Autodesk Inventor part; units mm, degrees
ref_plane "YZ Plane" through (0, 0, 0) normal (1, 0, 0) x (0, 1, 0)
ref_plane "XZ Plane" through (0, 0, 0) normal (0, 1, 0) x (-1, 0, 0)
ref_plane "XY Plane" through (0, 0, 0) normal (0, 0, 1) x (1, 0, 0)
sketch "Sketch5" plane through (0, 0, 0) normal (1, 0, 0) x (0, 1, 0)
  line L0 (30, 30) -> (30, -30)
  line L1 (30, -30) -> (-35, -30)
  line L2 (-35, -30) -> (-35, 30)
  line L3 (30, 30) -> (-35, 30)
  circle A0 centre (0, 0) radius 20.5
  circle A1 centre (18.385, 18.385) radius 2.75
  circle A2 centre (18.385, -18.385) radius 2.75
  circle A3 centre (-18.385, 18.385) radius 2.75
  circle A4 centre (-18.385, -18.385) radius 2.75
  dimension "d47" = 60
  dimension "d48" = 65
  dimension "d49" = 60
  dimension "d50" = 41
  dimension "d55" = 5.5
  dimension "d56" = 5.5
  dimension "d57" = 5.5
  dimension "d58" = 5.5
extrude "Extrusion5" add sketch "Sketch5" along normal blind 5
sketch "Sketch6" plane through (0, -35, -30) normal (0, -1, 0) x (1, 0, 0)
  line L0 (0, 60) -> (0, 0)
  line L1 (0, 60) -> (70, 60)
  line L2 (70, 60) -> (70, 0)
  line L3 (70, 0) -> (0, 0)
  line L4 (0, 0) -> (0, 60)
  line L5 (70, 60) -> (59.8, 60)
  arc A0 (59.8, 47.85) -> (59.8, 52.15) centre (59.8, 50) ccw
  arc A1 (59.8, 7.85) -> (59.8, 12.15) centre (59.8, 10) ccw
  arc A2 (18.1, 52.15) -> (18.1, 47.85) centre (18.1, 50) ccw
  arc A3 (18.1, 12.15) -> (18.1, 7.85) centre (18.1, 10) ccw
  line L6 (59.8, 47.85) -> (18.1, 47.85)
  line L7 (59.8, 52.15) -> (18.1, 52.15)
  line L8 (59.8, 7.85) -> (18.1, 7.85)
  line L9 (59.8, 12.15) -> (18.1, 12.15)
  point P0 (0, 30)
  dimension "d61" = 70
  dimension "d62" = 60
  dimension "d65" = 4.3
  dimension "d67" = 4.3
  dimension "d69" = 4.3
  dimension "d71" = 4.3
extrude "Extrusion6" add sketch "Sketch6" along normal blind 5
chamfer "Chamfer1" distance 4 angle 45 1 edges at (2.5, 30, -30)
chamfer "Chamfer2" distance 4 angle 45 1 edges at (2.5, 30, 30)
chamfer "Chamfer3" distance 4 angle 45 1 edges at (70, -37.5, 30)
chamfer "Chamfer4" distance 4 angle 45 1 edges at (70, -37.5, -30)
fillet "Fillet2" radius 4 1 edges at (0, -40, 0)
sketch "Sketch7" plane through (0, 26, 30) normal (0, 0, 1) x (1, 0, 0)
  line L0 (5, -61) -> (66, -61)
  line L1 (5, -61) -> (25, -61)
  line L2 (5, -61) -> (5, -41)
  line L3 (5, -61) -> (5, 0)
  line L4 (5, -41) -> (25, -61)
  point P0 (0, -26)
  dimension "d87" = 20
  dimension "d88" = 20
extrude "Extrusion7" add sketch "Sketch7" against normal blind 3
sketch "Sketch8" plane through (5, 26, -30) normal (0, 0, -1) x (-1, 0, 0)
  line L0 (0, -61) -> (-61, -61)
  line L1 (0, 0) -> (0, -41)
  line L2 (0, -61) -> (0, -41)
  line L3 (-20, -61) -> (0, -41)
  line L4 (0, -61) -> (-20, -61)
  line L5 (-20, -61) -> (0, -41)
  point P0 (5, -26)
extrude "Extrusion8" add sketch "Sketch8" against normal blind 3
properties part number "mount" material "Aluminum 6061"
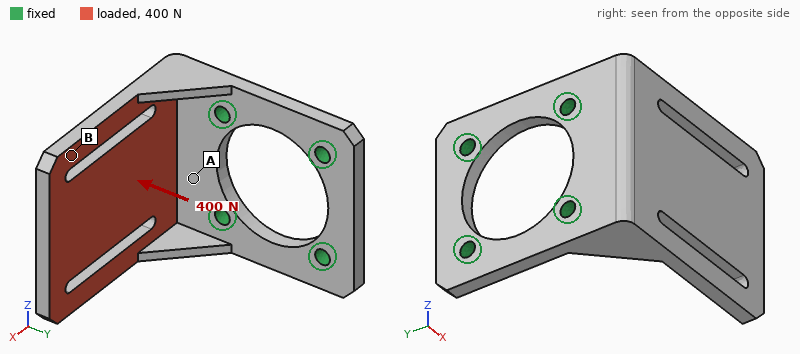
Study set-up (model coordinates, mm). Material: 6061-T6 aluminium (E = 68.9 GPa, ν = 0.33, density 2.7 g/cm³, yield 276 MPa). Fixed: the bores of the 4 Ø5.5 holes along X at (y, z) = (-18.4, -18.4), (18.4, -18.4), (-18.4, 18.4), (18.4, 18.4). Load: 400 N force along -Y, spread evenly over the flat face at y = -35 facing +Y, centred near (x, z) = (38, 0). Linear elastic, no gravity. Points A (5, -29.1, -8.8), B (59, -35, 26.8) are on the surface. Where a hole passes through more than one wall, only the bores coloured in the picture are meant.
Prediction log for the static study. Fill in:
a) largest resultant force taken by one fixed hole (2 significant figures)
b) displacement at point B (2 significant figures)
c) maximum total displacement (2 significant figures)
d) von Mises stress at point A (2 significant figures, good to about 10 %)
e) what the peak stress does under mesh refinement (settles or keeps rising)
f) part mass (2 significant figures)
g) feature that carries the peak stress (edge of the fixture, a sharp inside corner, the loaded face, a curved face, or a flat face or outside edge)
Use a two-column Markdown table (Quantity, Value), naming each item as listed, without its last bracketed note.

| Quantity | Value |
|---|---|
| largest resultant force taken by one fixed hole | 170 N |
| displacement at point B | 0.36 mm |
| maximum total displacement | 0.48 mm |
| von Mises stress at point A | 24 MPa |
| what the peak stress does under mesh refinement | keeps rising |
| part mass | 87 g |
| feature that carries the peak stress | edge of the fixture |
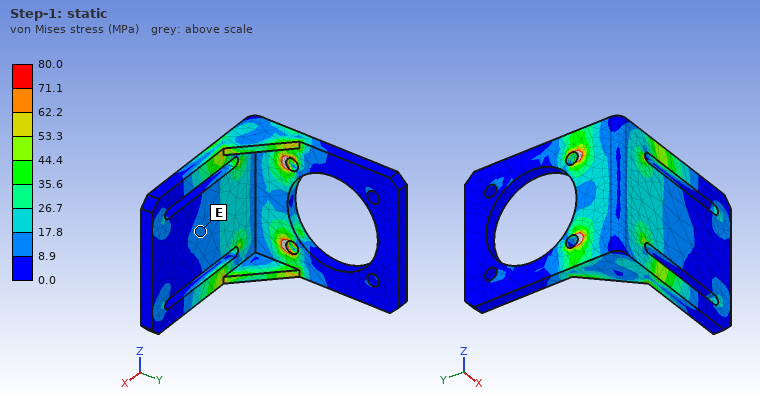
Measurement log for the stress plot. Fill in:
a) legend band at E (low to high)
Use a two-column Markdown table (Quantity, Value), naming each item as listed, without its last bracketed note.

| Quantity | Value |
|---|---|
| legend band at E | 8.9 to 17.8 MPa |
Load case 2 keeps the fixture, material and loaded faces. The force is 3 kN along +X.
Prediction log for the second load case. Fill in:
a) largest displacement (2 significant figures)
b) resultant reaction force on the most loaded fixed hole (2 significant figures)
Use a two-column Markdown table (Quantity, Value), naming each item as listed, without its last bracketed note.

| Quantity | Value |
|---|---|
| largest displacement | 0.34 mm |
| resultant reaction force on the most loaded fixed hole | 1.6 kN |
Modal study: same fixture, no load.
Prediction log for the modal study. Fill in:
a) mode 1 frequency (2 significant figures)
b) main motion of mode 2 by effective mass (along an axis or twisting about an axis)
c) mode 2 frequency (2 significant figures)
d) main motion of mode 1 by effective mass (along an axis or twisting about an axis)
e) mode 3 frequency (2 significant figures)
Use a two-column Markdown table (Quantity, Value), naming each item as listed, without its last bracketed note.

| Quantity | Value |
|---|---|
| mode 1 frequency | 840 Hz |
| main motion of mode 2 by effective mass | along Z |
| mode 2 frequency | 1800 Hz |
| main motion of mode 1 by effective mass | along Y |
| mode 3 frequency | 3100 Hz |
